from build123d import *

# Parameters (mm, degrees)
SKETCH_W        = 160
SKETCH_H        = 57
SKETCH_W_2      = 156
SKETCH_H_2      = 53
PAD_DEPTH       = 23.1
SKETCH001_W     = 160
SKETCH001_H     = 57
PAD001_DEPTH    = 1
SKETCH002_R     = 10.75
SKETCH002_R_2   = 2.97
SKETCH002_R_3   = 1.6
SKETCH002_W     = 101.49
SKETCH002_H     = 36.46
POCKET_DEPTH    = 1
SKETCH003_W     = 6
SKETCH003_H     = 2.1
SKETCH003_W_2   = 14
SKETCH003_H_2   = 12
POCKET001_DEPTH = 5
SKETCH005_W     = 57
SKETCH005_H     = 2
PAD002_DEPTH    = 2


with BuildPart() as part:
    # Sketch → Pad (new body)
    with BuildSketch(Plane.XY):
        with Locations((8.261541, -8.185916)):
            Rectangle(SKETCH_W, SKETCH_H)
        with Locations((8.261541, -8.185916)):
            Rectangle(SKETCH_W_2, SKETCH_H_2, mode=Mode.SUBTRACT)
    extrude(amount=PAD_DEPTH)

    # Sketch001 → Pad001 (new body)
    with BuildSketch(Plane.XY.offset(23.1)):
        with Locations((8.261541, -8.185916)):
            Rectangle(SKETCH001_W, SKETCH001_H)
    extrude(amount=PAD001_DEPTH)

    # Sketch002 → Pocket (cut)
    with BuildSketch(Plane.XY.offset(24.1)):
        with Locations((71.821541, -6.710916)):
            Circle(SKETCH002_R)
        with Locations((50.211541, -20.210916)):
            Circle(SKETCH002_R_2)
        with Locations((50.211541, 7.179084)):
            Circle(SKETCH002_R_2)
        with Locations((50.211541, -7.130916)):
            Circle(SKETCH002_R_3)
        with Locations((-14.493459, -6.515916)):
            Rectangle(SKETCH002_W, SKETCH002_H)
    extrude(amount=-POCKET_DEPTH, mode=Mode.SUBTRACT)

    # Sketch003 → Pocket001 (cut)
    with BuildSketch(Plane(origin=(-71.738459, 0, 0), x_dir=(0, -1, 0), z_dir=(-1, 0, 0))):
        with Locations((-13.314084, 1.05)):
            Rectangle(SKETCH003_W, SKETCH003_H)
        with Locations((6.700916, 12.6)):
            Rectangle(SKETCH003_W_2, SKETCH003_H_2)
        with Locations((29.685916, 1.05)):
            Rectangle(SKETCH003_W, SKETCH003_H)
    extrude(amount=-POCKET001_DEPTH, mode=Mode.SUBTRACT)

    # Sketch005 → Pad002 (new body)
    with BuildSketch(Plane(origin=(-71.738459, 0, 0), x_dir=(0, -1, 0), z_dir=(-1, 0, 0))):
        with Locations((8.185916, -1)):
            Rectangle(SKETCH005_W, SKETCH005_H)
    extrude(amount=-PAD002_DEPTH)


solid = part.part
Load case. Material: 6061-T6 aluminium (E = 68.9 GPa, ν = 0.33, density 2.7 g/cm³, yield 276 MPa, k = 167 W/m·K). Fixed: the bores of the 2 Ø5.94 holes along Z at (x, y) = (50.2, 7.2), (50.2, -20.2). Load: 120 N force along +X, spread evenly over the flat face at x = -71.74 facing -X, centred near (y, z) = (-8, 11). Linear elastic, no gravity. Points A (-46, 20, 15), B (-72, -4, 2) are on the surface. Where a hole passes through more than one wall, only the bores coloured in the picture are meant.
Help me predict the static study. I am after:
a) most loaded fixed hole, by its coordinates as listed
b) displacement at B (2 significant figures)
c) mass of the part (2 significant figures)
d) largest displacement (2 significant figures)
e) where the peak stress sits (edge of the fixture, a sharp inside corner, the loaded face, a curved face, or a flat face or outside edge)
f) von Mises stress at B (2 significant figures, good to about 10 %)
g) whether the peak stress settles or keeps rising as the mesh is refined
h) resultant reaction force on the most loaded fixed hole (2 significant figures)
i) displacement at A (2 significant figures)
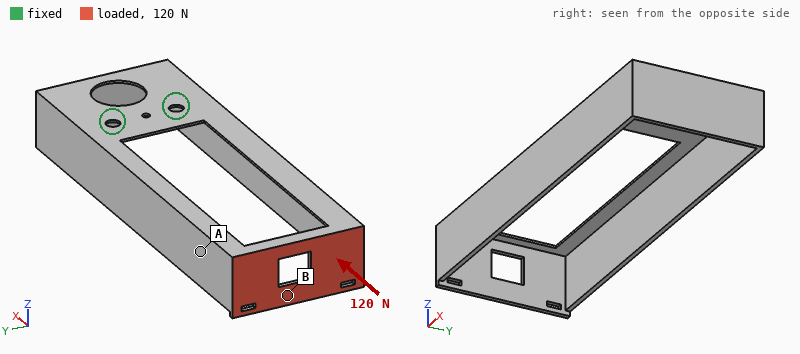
(50.2, -20.2)
1.8 mm
66 g
1.8 mm
edge of the fixture
18 MPa
keeps rising
67 N
1.4 mm
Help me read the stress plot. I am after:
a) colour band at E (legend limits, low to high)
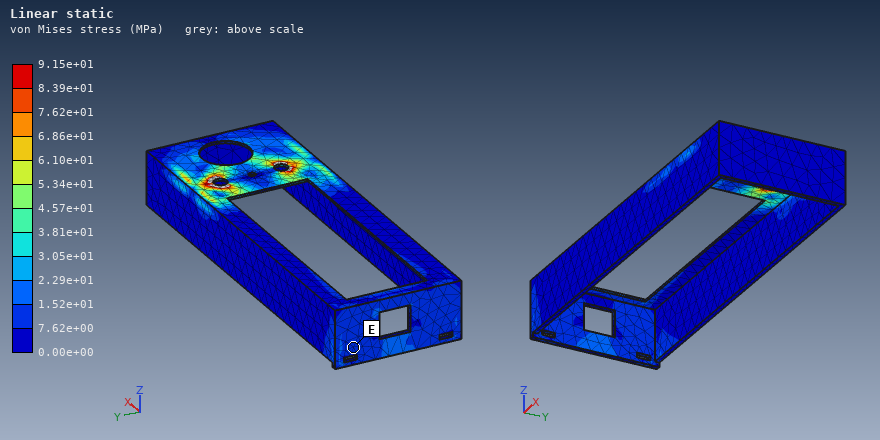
7.62e+00 to 1.52e+01 MPa
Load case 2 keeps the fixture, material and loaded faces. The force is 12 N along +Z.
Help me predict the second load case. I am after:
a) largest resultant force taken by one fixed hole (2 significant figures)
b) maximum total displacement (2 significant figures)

6.7 N
1.8 mm
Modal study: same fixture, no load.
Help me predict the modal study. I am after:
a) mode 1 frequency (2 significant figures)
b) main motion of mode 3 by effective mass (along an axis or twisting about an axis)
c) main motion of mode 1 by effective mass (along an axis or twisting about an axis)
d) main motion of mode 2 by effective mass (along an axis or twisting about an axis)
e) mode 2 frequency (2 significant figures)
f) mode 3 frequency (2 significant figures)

92 Hz
along Y
along Z
along Y
280 Hz
480 Hz
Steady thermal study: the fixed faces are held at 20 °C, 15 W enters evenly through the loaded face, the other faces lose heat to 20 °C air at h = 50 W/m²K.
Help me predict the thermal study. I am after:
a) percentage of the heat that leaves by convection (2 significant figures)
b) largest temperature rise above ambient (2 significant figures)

92 %
39 K
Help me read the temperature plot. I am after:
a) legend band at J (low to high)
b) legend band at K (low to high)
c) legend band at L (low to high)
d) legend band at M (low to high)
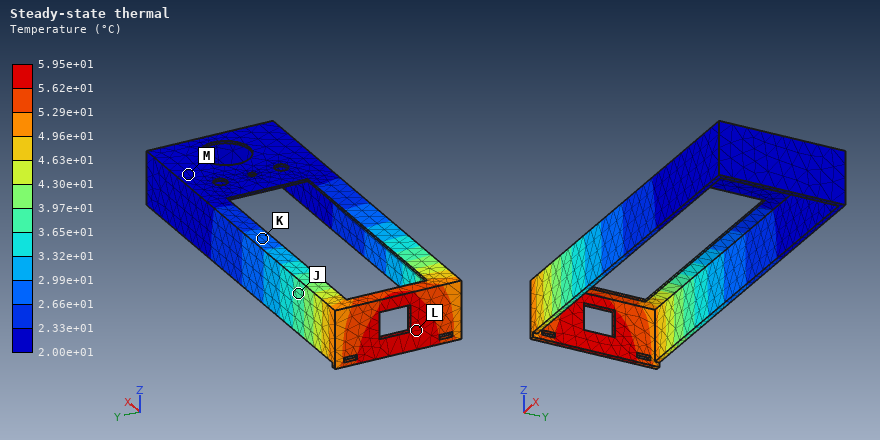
3.65e+01 to 3.97e+01 °C
2.66e+01 to 2.99e+01 °C
5.62e+01 to 5.95e+01 °C
2.00e+01 to 2.33e+01 °C
